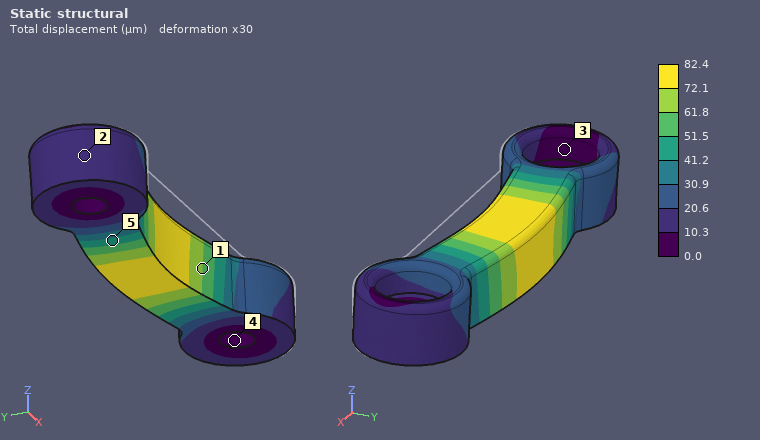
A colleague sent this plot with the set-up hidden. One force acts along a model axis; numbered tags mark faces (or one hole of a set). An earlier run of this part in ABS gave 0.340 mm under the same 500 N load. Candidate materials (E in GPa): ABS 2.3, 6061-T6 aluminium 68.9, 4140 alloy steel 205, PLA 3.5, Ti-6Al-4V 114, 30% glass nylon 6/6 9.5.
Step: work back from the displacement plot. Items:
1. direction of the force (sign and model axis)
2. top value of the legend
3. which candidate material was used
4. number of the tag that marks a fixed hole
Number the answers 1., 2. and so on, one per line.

1. +Y
2. 82.4 µm
3. 30% glass nylon 6/6
4. 4
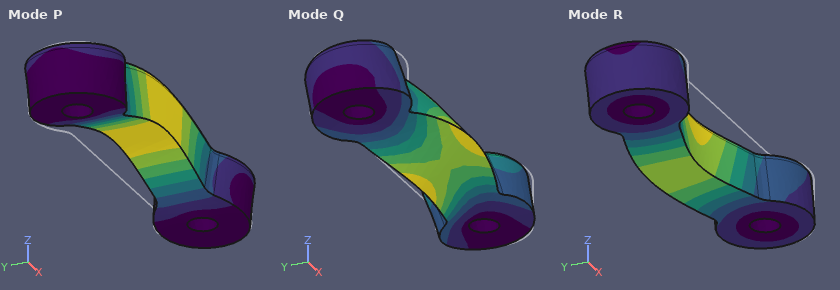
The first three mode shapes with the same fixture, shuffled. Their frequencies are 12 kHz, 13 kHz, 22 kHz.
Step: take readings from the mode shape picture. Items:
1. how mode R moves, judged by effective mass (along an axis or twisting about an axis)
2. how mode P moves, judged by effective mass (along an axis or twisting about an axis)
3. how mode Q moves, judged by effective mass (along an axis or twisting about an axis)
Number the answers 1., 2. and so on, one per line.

1. along Y
2. along Z
3. twisting about X
